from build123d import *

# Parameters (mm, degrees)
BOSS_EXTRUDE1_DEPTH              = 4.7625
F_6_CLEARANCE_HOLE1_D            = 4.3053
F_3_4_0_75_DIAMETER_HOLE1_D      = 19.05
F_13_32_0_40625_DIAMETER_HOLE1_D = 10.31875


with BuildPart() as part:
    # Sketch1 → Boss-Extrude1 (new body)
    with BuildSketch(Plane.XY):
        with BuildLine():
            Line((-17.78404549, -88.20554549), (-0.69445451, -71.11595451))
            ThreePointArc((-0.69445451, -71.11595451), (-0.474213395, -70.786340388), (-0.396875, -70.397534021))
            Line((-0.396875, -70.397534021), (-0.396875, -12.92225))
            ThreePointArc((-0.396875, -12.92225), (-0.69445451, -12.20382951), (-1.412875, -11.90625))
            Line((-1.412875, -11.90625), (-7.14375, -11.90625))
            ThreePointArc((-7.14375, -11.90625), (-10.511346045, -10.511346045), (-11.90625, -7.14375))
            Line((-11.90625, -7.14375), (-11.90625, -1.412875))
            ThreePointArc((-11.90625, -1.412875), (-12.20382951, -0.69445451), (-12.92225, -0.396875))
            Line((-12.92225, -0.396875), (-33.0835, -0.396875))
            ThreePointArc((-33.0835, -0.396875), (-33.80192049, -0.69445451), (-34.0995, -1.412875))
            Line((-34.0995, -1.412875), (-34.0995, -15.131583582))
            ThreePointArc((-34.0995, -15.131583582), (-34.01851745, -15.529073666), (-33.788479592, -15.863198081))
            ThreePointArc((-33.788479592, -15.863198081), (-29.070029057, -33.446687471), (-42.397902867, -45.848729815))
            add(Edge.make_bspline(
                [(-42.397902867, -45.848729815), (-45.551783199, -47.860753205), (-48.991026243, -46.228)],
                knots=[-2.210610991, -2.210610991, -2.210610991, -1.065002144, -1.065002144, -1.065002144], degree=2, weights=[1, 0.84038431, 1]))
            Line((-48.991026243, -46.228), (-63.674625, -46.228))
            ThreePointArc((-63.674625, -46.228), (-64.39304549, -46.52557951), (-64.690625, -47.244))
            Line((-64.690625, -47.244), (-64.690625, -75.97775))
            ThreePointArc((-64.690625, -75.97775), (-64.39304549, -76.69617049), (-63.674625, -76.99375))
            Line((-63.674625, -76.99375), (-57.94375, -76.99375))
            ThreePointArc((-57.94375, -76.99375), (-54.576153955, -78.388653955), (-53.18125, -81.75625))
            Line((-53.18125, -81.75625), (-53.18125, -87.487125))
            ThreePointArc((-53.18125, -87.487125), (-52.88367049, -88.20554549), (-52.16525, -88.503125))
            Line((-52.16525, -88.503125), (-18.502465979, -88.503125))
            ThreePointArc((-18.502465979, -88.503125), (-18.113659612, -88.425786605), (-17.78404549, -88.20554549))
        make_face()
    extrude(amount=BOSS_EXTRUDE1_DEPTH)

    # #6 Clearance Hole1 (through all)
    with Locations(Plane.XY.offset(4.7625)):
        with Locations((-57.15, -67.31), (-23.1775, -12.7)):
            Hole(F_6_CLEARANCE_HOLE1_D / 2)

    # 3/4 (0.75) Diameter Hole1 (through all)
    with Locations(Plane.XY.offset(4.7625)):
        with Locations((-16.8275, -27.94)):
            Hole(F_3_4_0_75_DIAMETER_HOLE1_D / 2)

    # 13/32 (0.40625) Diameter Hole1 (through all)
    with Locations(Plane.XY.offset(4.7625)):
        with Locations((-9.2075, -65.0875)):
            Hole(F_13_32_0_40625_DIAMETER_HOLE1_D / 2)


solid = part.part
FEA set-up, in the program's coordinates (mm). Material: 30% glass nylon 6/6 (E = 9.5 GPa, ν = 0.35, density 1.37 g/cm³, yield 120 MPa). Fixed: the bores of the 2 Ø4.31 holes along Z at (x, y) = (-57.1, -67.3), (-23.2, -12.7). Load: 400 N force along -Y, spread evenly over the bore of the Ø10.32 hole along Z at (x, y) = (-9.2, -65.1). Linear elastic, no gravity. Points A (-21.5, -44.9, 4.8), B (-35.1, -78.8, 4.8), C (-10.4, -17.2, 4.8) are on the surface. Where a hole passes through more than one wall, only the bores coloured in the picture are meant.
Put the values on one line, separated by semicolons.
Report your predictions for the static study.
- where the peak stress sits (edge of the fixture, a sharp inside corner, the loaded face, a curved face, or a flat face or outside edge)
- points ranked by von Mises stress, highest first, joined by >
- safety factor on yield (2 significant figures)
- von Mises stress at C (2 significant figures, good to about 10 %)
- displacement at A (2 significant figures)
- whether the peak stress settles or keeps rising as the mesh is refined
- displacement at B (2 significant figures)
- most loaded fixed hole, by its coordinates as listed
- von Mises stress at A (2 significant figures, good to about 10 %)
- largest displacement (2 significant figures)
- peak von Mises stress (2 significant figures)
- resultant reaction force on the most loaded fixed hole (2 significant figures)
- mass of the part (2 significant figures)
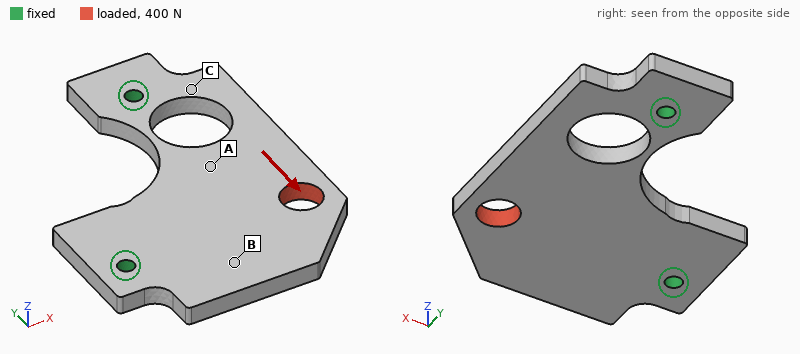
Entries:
a curved face; C > A > B; 4.0; 7.3 MPa; 38 µm; settles; 27 µm; (-23.2, -12.7); 4.3 MPa; 61 µm; 30 MPa; 370 N; 22 g
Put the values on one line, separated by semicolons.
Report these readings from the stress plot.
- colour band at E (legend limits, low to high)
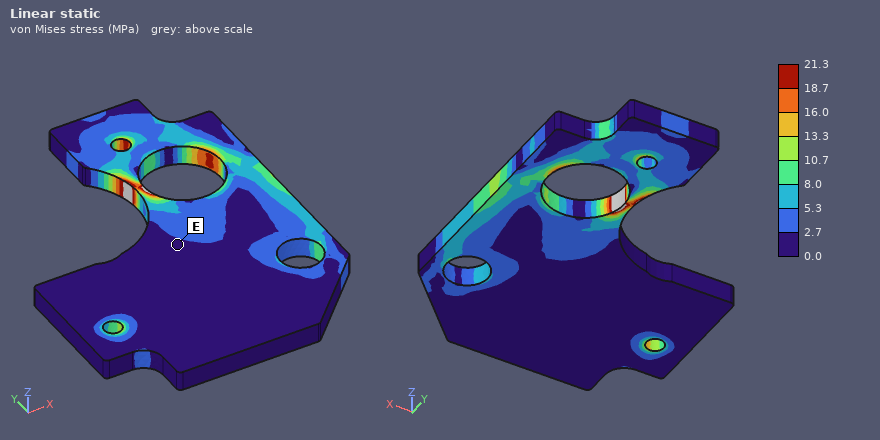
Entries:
0.0 to 2.7 MPa
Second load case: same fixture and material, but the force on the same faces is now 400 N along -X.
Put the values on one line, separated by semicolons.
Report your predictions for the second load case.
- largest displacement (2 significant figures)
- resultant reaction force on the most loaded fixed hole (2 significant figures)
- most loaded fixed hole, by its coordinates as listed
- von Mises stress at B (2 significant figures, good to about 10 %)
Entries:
25 µm; 390 N; (-57.1, -67.3); 2.0 MPa
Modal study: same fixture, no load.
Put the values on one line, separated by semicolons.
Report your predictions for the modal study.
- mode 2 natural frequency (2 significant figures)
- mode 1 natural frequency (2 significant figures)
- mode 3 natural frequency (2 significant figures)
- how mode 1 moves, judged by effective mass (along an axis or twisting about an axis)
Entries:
2100 Hz; 800 Hz; 3400 Hz; along Z
